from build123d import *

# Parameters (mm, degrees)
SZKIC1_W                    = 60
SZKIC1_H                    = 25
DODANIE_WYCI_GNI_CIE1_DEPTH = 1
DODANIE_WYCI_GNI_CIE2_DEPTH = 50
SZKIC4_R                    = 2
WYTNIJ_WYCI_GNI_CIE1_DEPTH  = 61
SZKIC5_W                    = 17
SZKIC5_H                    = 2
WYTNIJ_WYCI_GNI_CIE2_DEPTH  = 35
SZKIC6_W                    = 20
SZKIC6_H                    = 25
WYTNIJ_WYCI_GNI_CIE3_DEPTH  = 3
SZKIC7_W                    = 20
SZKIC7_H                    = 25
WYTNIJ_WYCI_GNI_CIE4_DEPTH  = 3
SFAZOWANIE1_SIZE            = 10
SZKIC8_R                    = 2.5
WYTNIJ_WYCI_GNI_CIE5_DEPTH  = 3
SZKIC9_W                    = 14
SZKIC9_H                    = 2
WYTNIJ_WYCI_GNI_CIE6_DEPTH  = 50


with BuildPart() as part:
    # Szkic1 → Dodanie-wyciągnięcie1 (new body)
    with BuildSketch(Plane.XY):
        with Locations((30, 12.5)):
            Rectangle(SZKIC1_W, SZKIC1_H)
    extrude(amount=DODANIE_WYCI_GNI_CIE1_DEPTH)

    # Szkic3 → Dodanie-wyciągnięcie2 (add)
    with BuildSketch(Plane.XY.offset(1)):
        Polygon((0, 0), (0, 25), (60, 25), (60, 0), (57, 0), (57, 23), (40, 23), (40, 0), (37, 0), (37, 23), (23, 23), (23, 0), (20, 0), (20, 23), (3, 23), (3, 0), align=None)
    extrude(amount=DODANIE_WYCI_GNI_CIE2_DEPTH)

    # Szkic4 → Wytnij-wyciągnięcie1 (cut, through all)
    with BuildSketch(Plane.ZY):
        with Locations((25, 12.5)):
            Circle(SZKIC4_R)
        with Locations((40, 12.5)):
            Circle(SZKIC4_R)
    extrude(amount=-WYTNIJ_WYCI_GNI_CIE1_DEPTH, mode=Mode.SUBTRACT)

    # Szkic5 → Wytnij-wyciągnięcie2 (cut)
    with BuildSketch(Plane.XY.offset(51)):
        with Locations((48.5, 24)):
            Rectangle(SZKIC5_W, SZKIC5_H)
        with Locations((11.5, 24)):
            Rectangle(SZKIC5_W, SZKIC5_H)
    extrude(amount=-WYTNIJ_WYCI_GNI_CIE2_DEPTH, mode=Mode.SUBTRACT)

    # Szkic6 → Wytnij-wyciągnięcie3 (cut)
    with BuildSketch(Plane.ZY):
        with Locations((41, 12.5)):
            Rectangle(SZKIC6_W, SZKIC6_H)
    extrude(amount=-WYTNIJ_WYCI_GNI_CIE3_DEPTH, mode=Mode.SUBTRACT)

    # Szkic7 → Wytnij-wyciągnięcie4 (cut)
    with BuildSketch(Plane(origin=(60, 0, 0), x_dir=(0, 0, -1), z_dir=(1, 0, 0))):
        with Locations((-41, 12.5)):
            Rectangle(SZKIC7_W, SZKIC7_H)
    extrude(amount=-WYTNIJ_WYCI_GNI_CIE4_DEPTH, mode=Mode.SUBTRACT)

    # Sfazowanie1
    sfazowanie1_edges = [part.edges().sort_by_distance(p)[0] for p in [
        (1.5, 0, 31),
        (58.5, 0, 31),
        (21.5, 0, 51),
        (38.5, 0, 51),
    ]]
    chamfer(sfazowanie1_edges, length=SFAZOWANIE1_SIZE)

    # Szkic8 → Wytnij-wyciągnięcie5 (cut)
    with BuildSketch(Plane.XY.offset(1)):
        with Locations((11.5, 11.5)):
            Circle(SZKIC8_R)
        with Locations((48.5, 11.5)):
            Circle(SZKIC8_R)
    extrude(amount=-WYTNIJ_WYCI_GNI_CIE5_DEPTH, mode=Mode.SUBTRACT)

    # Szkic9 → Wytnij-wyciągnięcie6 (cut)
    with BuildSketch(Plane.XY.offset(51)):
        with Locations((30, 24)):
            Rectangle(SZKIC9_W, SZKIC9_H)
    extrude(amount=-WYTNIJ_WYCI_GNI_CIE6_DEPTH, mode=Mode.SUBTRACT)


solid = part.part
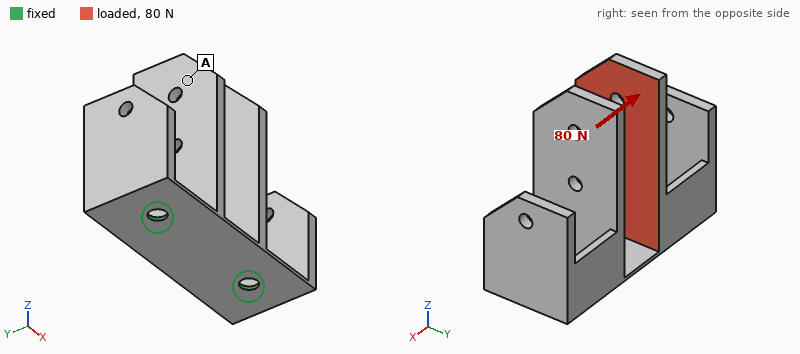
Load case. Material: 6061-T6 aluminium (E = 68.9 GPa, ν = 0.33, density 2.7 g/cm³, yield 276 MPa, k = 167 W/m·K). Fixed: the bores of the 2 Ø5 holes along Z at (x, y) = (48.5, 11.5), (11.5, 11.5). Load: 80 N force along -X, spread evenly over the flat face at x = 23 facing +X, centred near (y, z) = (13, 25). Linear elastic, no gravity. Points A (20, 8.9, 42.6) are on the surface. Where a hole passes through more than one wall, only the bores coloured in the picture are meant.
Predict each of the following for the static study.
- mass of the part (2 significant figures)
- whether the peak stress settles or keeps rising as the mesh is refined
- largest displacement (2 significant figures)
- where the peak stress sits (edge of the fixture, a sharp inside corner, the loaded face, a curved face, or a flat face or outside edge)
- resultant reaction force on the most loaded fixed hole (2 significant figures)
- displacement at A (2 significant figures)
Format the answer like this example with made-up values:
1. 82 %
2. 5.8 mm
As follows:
1. 37 g
2. keeps rising
3. 0.81 mm
4. edge of the fixture
5. 64 N
6. 0.66 mm
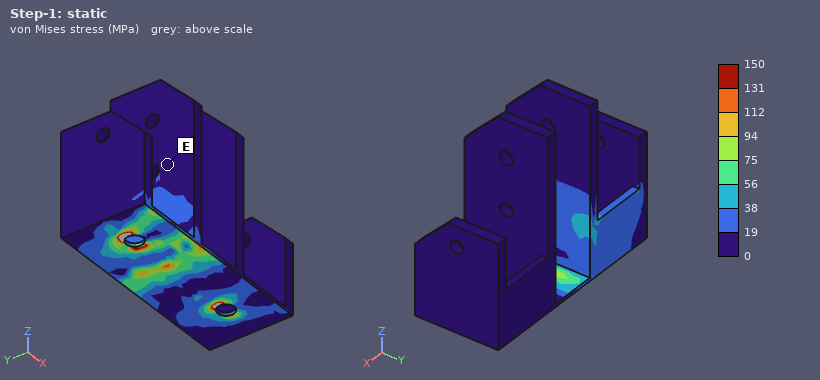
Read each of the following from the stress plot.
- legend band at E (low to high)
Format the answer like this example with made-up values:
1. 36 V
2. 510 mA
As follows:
1. 0 to 19 MPa
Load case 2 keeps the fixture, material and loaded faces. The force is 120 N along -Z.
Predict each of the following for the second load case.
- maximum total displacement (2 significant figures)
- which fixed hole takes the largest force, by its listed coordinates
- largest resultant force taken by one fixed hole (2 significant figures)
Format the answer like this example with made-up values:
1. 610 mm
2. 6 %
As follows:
1. 0.34 mm
2. (11.5, 11.5)
3. 93 N
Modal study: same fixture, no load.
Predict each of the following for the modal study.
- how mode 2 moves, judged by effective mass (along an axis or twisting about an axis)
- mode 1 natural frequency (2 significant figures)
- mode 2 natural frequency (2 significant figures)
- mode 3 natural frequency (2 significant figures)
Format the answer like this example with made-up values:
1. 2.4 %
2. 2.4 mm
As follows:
1. along Y
2. 470 Hz
3. 530 Hz
4. 740 Hz
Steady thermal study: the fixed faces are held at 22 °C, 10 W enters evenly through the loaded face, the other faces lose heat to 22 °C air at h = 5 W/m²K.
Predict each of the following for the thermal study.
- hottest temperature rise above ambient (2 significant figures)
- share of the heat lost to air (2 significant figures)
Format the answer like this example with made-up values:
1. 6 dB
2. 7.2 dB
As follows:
1. 31 K
2. 4.8 %
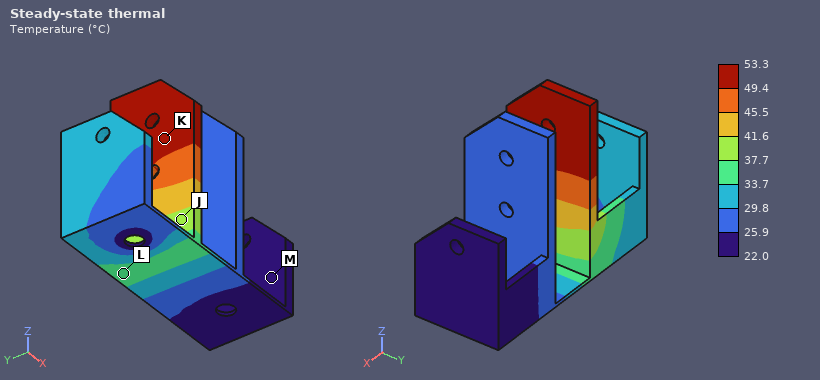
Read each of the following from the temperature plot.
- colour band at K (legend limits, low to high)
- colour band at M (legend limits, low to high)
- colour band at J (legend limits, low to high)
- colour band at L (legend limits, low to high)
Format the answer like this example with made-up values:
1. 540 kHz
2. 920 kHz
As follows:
1. 49.4 to 53.3 °C
2. 22.0 to 25.9 °C
3. 37.7 to 41.6 °C
4. 33.7 to 37.7 °C
